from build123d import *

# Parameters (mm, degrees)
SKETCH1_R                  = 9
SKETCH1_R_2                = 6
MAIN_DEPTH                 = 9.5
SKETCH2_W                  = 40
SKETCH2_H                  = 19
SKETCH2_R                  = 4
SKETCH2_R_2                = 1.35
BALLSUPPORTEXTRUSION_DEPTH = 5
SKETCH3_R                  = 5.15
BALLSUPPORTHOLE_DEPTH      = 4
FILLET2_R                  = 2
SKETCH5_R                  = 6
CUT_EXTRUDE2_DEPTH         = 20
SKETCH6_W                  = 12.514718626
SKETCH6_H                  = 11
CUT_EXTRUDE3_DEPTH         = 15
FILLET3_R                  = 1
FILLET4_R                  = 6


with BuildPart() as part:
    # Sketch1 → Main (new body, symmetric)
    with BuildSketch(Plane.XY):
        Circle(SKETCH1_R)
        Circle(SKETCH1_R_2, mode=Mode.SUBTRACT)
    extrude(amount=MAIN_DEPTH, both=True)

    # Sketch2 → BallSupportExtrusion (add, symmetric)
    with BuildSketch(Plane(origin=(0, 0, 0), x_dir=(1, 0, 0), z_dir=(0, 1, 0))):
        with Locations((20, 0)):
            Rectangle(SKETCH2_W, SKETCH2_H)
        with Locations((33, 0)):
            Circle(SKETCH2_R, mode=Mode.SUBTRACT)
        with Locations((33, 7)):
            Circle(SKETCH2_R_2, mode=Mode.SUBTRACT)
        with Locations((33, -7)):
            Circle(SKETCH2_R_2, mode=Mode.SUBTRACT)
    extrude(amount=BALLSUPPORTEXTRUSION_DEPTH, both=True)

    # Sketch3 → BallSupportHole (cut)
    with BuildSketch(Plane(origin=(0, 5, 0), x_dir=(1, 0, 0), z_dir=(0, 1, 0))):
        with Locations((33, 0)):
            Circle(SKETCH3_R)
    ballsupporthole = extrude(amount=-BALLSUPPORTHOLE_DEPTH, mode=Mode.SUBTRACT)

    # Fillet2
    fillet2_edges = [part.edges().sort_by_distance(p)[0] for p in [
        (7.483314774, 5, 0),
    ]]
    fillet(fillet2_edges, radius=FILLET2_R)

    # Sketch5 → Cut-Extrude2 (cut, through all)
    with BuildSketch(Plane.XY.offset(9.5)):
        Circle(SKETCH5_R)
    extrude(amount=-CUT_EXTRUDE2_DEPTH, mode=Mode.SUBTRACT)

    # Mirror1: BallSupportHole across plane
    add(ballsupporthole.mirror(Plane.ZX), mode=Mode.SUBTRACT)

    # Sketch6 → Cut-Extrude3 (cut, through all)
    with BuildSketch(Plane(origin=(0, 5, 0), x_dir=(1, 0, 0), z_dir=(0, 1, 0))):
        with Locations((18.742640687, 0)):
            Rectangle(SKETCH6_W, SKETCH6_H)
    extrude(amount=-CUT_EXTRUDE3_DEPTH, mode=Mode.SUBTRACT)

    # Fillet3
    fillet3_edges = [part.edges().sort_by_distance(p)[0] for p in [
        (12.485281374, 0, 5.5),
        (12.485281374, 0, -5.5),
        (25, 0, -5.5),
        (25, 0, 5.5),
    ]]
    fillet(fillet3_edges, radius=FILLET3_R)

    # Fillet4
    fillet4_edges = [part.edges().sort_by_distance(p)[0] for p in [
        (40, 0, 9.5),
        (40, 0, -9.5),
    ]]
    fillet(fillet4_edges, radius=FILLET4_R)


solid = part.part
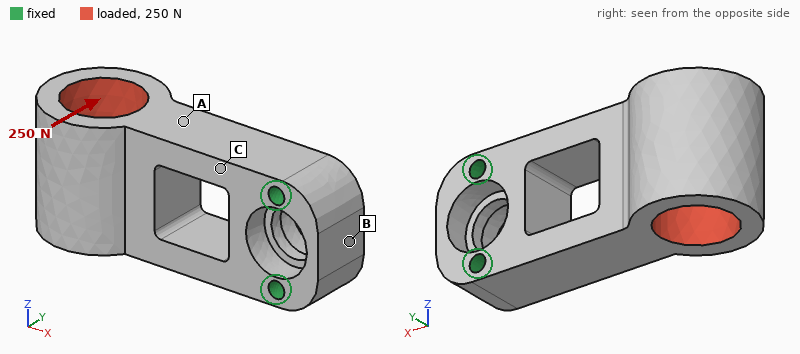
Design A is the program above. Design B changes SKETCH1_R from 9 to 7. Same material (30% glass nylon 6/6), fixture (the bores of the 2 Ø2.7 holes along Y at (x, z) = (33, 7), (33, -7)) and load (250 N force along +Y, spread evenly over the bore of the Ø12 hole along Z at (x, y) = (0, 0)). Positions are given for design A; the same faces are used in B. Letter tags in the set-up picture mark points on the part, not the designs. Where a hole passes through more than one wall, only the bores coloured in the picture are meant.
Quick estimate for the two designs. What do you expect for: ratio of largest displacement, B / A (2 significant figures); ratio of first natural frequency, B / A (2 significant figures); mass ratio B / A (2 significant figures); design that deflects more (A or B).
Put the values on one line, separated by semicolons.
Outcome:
1.6; 1.4; 0.76; B
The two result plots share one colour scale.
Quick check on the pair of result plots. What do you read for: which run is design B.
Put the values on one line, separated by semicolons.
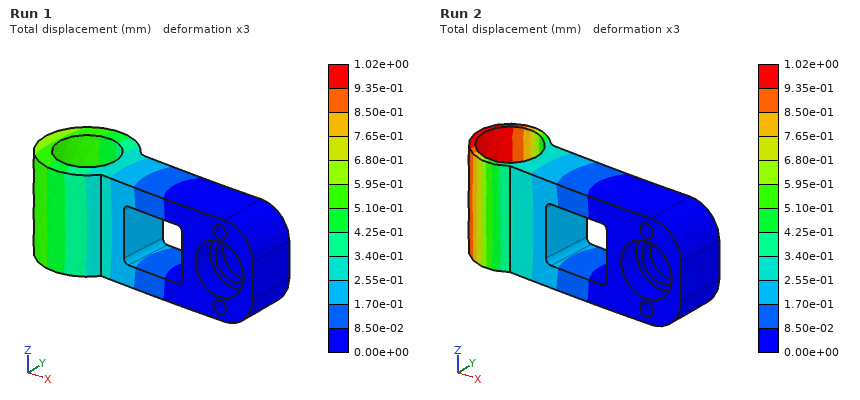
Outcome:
Run 2
